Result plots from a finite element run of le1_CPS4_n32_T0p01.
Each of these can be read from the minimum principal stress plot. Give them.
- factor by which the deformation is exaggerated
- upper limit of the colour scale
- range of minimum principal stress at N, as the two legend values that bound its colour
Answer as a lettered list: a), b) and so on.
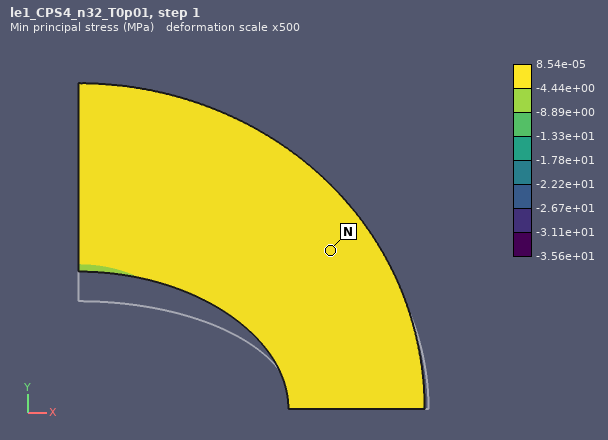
a) 500
b) 8.54e-05 MPa
c) -4.44e+00 to 8.54e-05 MPa
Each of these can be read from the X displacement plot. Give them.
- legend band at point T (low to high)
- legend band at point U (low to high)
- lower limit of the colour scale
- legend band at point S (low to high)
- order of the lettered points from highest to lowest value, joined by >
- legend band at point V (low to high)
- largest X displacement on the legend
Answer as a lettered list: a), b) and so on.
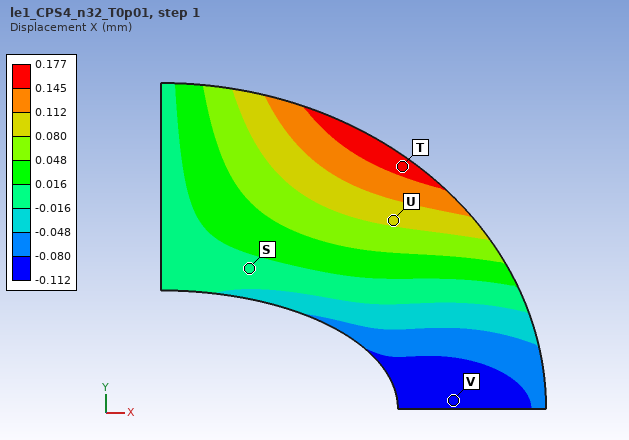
a) 0.145 to 0.177 mm
b) 0.080 to 0.112 mm
c) -0.112 mm
d) -0.016 to 0.016 mm
e) T > U > S > V
f) -0.112 to -0.080 mm
g) 0.177 mm
